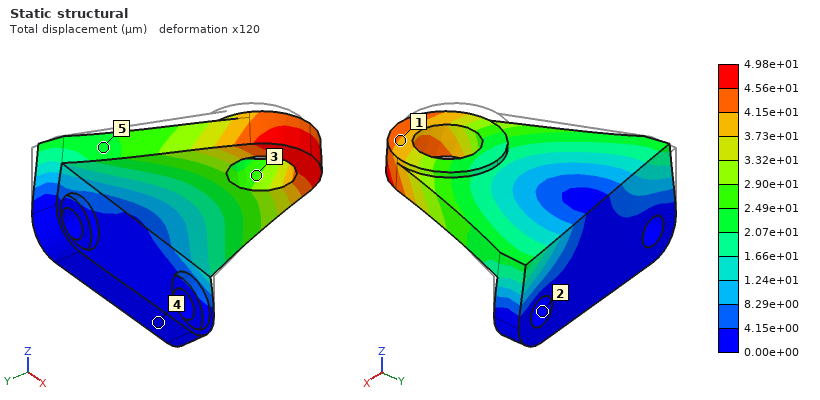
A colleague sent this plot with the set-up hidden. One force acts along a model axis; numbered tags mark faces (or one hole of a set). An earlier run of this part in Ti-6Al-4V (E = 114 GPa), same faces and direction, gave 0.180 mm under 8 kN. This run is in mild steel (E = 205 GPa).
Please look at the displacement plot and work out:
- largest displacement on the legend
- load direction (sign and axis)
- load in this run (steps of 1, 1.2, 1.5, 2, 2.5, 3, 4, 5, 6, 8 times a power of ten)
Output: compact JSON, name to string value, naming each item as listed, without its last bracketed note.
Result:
{"largest displacement on the legend": "4.98e+01 µm", "load direction": "+X", "load in this run": "4 kN"}
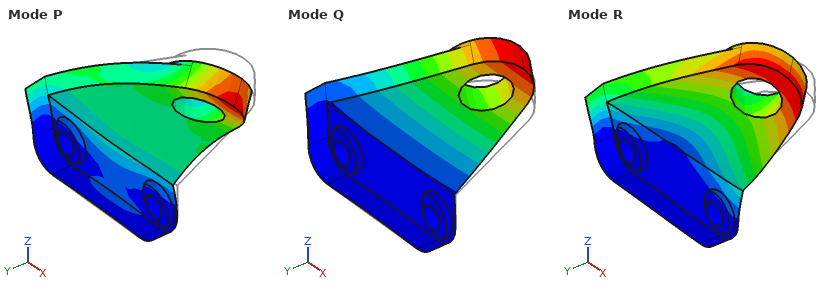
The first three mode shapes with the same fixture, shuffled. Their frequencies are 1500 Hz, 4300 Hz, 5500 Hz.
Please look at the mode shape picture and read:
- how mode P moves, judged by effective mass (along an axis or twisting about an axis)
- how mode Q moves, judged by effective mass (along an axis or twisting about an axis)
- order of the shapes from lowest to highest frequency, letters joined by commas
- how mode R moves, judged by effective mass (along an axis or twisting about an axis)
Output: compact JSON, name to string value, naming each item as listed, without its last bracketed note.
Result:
{"how mode P moves, judged by effective mass": "along Y", "how mode Q moves, judged by effective mass": "along Z", "order of the shapes from lowest to highest frequency, letters joined by commas": "Q, R, P", "how mode R moves, judged by effective mass": "along X"}
